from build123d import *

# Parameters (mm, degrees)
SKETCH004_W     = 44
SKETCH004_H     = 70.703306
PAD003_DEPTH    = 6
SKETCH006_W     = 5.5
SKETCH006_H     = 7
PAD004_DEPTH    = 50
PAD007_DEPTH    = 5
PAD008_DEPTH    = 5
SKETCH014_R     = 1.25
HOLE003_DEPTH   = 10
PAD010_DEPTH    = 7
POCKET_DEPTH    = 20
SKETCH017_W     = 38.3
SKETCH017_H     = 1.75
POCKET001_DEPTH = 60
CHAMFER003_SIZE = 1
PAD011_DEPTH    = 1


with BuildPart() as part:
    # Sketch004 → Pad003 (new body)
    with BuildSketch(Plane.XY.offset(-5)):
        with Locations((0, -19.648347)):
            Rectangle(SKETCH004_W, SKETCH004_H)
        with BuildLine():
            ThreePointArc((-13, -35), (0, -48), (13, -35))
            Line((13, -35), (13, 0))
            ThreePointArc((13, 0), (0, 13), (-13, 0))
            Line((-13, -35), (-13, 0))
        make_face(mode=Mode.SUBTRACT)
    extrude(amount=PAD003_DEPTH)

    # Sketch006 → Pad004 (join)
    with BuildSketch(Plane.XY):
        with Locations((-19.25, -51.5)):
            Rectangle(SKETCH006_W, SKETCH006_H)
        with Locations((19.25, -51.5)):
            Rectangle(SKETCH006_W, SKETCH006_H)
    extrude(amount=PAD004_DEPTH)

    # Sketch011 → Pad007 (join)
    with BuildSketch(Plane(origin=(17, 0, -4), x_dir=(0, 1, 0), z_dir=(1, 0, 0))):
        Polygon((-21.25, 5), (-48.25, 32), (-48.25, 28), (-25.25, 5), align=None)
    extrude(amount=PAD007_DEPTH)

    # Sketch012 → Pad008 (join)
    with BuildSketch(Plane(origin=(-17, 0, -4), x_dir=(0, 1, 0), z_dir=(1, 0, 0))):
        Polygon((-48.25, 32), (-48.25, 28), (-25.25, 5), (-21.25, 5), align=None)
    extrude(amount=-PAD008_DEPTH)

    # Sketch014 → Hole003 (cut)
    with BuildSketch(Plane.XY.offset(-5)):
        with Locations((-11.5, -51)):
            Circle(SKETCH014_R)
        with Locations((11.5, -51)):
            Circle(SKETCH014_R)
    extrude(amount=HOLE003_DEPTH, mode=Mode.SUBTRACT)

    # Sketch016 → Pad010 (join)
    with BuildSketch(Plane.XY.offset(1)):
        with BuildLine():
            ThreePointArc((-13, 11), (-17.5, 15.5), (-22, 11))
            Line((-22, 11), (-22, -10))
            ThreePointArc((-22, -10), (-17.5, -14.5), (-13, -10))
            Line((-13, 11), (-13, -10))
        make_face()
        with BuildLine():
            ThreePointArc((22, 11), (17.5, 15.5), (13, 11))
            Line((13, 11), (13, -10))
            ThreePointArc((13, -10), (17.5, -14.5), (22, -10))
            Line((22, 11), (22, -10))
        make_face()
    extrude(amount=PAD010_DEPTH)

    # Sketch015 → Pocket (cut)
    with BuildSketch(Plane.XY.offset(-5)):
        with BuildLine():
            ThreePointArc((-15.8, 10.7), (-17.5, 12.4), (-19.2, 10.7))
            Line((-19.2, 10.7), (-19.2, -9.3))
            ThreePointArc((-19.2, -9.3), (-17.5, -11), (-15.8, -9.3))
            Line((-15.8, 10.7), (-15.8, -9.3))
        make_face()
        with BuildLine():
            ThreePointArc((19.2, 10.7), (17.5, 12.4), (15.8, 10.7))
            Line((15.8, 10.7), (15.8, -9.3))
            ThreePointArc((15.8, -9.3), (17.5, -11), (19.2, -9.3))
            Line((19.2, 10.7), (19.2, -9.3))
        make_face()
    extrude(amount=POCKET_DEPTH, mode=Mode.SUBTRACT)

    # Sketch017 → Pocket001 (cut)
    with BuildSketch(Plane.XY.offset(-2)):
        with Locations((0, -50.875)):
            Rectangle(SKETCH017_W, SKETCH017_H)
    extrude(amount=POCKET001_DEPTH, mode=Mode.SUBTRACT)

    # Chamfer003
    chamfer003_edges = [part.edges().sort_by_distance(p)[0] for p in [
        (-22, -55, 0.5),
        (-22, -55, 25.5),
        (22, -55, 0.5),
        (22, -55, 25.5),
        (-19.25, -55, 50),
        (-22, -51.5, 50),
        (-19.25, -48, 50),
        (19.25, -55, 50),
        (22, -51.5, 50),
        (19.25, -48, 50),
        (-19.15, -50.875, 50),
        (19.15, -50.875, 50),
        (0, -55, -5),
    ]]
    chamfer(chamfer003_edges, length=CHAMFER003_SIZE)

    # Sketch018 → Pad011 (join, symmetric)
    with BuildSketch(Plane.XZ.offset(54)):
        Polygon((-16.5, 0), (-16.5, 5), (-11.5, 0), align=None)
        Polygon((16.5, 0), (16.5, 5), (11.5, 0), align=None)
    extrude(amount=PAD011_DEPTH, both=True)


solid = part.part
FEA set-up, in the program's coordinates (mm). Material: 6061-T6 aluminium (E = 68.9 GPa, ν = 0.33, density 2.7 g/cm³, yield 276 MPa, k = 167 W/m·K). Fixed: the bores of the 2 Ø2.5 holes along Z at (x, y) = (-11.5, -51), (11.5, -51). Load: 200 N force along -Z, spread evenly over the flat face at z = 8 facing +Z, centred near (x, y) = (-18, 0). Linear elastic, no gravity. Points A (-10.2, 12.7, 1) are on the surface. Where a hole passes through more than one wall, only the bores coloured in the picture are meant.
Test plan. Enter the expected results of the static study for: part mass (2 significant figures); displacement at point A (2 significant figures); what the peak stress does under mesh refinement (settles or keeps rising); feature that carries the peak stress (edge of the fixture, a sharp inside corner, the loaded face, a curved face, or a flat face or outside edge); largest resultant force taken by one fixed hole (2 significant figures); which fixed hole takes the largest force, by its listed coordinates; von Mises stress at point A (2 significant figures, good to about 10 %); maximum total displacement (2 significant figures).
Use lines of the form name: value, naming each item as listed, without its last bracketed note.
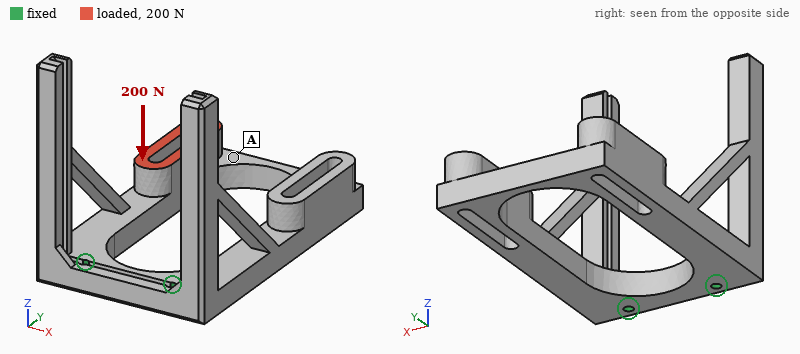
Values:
part mass: 42 g
displacement at point A: 0.47 mm
what the peak stress does under mesh refinement: keeps rising
feature that carries the peak stress: edge of the fixture
largest resultant force taken by one fixed hole: 190 N
which fixed hole takes the largest force, by its listed coordinates: (-11.5, -51)
von Mises stress at point A: 15 MPa
maximum total displacement: 0.57 mm
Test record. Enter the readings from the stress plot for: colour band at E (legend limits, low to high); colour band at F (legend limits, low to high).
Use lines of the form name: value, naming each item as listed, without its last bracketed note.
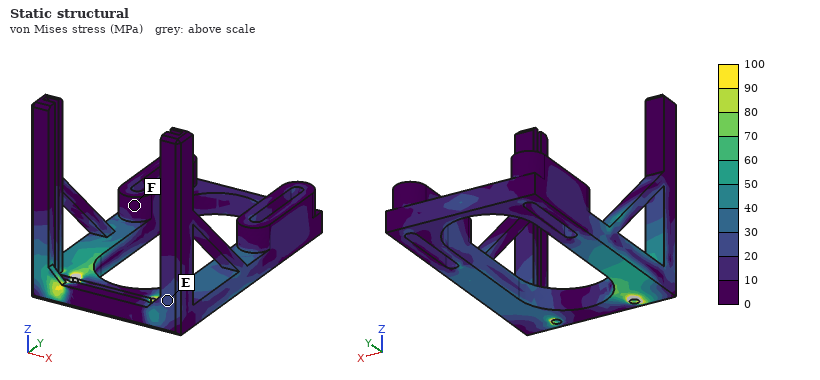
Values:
colour band at E: 20 to 30 MPa
colour band at F: 0 to 10 MPa
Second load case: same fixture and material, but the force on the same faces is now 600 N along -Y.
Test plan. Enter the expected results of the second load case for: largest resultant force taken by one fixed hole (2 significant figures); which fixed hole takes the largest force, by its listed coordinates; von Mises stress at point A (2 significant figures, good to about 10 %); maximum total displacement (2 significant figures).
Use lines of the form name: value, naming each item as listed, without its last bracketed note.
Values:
largest resultant force taken by one fixed hole: 700 N
which fixed hole takes the largest force, by its listed coordinates: (-11.5, -51)
von Mises stress at point A: 15 MPa
maximum total displacement: 0.50 mm
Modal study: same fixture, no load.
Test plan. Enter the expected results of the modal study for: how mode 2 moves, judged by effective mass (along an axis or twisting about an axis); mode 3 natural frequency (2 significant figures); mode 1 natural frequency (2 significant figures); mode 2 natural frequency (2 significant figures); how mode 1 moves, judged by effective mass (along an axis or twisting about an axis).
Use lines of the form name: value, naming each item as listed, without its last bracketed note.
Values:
how mode 2 moves, judged by effective mass: along X
mode 3 natural frequency: 1600 Hz
mode 1 natural frequency: 890 Hz
mode 2 natural frequency: 1600 Hz
how mode 1 moves, judged by effective mass: along Z
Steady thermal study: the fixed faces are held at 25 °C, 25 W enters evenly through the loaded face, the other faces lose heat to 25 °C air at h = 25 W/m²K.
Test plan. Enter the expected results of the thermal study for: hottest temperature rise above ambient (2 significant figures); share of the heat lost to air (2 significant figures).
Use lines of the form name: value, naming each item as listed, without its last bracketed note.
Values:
hottest temperature rise above ambient: 77 K
share of the heat lost to air: 27 %
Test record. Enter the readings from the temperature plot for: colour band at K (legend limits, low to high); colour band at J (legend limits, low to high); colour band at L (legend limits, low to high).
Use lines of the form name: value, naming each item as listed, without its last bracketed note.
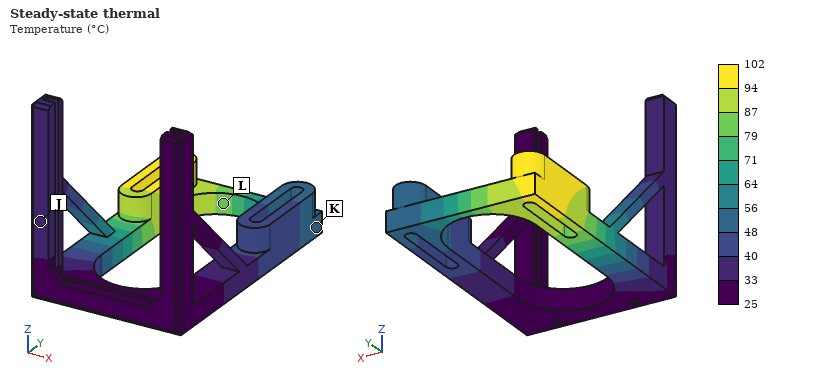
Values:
colour band at K: 48 to 56 °C
colour band at J: 33 to 40 °C
colour band at L: 79 to 87 °C
